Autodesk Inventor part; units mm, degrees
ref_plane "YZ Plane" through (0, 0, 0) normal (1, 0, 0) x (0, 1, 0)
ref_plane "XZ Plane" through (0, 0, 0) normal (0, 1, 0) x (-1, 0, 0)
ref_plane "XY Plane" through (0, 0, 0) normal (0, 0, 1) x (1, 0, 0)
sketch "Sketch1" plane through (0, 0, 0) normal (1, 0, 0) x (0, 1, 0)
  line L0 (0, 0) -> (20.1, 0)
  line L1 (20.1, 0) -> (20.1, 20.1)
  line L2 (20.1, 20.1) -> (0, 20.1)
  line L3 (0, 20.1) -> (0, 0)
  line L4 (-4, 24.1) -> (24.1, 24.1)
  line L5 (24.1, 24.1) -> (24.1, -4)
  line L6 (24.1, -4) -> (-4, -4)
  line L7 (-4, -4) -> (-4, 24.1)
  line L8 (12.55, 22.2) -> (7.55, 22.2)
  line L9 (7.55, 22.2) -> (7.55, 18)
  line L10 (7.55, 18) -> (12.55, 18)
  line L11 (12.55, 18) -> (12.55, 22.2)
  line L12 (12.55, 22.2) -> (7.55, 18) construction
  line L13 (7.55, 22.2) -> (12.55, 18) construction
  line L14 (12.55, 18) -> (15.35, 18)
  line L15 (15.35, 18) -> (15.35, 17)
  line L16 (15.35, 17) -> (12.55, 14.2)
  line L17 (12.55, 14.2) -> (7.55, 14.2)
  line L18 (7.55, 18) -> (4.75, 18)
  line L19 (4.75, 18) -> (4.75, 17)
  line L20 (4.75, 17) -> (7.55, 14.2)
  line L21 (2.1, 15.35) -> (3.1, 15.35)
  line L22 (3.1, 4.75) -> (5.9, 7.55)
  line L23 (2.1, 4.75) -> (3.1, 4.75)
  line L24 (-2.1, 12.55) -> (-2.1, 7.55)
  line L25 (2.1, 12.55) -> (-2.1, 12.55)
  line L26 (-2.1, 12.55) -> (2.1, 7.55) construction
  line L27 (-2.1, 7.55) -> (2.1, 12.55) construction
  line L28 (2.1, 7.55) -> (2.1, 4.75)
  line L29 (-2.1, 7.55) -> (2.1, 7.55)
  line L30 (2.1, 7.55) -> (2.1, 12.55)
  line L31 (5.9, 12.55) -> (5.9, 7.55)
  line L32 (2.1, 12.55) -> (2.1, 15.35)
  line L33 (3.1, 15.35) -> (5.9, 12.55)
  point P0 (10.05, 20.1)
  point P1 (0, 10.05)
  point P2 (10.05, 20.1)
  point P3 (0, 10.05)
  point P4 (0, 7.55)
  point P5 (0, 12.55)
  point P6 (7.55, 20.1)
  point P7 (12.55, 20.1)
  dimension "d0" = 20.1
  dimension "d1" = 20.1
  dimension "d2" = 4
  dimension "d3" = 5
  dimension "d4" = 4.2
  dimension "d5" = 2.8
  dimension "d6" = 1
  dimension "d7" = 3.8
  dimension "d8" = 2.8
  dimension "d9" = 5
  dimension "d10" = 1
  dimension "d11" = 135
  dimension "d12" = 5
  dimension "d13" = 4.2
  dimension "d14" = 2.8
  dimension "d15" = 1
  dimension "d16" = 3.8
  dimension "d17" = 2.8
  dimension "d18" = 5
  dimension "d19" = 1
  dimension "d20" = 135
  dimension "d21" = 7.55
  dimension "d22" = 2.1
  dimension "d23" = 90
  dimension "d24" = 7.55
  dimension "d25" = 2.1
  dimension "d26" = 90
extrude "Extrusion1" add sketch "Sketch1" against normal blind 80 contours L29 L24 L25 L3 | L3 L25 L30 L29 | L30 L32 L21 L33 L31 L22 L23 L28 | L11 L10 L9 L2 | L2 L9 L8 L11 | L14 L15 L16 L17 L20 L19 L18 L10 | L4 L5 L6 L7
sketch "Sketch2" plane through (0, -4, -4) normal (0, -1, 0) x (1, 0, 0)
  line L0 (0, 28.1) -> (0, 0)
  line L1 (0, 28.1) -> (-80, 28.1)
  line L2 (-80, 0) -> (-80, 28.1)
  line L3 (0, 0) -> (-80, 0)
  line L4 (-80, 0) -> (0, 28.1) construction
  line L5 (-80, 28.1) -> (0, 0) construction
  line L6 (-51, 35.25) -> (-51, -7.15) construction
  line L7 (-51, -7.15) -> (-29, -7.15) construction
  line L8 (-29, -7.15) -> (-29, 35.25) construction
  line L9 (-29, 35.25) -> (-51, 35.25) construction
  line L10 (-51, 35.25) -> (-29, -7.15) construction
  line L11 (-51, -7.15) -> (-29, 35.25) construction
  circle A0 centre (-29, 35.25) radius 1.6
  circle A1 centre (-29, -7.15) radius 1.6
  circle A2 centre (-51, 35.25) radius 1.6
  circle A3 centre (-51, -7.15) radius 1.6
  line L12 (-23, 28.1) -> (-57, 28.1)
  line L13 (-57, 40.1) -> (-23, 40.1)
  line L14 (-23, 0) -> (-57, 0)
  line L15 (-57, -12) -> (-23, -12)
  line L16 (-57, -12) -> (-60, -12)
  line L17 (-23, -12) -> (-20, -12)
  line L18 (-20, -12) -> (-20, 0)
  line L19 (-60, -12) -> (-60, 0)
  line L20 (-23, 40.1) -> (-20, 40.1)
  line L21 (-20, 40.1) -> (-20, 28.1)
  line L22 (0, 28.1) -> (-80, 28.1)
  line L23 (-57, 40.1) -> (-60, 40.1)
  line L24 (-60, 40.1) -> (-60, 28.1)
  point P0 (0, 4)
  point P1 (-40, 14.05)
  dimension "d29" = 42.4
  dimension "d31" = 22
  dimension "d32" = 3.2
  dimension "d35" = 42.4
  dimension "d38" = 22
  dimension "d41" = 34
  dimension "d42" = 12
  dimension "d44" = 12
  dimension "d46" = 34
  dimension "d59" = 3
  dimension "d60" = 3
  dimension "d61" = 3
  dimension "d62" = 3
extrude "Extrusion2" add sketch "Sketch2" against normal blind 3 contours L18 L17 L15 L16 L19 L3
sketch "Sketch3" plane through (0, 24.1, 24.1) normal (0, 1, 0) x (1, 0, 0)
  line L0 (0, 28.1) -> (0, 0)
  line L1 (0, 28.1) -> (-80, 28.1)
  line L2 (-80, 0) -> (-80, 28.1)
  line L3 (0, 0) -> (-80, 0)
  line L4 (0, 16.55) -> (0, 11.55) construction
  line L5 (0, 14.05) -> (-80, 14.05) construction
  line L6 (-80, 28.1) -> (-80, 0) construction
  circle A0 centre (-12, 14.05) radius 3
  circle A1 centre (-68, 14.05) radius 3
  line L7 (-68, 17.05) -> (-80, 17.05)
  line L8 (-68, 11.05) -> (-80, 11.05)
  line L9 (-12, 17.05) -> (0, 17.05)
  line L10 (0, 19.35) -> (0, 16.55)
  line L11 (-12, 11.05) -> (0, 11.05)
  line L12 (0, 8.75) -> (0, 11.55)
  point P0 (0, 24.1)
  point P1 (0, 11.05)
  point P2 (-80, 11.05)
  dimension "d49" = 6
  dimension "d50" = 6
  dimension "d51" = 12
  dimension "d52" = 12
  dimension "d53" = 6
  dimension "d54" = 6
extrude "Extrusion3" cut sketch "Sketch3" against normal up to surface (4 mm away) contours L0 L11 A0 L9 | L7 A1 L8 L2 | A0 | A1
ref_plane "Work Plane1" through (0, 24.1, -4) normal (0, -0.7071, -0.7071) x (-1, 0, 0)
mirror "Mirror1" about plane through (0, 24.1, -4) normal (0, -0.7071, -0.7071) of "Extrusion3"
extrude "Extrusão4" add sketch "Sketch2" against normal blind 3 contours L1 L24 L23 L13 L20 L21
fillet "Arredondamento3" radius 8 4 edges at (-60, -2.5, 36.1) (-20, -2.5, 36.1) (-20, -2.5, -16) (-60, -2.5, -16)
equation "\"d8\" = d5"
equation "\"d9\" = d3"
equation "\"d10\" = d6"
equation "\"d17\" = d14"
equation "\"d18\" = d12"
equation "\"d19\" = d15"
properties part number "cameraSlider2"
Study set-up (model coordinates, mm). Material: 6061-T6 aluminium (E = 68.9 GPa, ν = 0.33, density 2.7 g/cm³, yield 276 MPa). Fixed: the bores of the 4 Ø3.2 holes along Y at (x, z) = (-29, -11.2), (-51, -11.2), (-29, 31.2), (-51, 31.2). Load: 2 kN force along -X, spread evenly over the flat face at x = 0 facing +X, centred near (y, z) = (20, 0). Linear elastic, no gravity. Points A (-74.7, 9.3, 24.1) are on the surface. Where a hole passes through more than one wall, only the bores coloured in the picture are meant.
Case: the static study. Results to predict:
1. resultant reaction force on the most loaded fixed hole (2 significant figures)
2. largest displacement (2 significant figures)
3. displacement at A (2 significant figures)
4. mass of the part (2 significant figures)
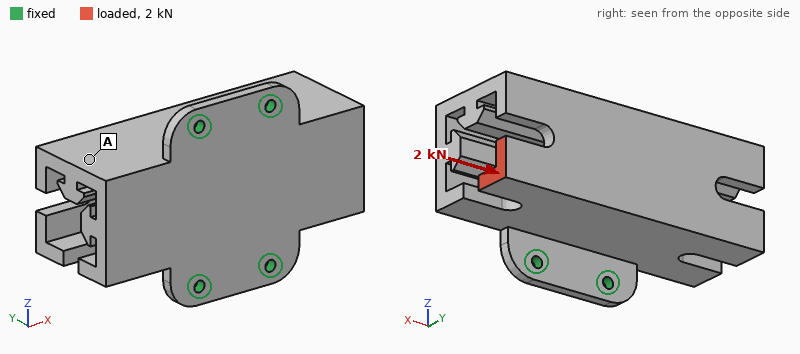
1.2 kN
0.17 mm
0.10 mm
110 g
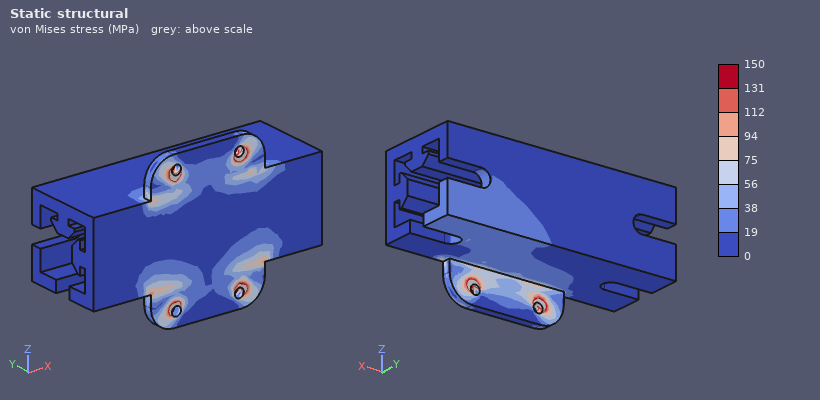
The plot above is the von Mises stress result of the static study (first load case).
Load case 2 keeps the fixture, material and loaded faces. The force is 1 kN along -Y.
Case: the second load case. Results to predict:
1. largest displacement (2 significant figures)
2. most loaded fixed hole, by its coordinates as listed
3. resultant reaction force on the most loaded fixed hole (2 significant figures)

0.25 mm
(-29, -11.2)
1.3 kN
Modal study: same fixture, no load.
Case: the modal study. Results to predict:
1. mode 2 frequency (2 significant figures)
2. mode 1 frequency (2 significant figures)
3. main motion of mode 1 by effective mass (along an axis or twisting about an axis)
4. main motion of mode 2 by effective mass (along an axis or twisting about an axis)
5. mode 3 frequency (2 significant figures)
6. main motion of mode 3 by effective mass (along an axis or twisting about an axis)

3900 Hz
2300 Hz
along X
along Z
4900 Hz
along Y
